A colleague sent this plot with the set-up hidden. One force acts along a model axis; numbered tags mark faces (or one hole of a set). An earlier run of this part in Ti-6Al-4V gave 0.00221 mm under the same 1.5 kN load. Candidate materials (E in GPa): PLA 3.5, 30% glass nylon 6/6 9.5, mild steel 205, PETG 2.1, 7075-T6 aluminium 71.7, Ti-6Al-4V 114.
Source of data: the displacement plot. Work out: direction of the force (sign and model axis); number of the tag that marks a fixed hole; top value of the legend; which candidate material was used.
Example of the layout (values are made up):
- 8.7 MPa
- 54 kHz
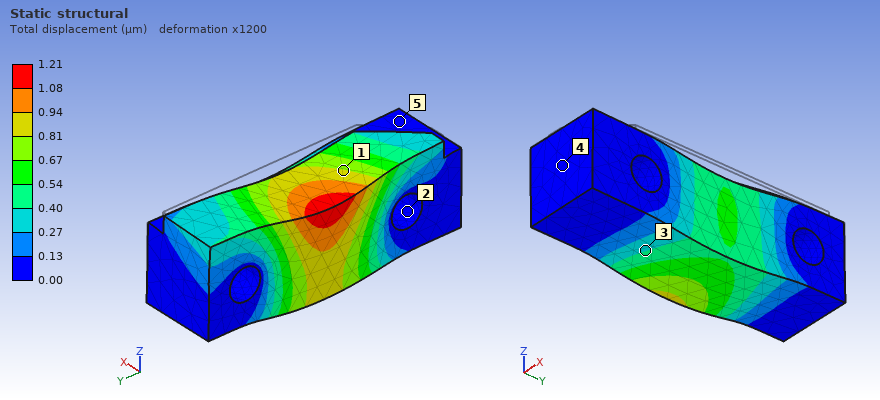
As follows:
- -Z
- 2
- 1.21 µm
- mild steel
